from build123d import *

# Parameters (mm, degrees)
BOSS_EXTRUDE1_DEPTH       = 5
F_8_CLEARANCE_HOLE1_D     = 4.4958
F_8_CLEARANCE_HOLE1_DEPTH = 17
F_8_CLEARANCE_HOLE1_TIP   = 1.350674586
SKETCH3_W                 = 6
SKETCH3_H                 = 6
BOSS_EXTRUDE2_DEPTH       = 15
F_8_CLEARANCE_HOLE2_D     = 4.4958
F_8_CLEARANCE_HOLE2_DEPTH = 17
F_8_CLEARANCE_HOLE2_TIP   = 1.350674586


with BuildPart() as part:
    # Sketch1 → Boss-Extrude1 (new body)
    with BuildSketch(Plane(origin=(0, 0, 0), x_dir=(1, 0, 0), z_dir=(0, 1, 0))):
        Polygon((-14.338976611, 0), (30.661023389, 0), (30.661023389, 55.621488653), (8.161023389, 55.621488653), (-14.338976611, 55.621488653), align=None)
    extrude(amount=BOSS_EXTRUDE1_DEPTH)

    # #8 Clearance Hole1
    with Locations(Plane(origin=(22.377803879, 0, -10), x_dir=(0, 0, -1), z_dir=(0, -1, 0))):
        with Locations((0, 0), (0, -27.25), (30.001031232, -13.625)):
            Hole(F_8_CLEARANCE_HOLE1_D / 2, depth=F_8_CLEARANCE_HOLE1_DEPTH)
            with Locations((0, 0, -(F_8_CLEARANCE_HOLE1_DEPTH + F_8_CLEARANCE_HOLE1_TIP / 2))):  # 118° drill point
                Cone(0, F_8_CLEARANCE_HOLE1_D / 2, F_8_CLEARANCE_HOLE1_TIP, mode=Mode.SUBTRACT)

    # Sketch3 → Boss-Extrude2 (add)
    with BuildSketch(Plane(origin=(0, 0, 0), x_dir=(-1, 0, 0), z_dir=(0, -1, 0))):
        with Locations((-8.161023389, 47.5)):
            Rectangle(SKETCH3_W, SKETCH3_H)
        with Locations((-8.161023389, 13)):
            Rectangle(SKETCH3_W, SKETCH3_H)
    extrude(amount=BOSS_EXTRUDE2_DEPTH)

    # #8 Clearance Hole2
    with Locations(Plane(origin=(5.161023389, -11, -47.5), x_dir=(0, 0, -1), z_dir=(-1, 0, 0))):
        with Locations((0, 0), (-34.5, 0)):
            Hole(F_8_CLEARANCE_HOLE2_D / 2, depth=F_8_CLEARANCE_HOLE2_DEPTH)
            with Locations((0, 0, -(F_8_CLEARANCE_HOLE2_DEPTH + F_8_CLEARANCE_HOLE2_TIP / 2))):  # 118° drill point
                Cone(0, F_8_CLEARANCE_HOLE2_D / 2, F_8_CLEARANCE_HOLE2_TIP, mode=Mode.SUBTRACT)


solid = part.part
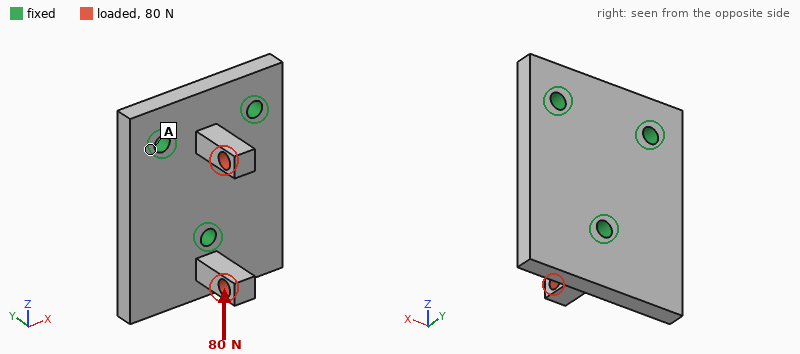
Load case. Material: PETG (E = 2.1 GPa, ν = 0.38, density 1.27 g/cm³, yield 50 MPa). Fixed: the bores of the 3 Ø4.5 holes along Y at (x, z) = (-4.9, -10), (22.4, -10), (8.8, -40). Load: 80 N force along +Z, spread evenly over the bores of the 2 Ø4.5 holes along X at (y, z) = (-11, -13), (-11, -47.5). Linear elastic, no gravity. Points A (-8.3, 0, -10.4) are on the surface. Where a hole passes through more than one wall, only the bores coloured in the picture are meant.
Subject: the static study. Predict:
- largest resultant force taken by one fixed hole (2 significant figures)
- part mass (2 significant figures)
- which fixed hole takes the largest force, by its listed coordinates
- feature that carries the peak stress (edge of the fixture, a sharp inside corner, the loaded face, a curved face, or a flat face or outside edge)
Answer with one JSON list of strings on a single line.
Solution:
["52 N", "17 g", "(8.8, -40)", "a flat face or outside edge"]
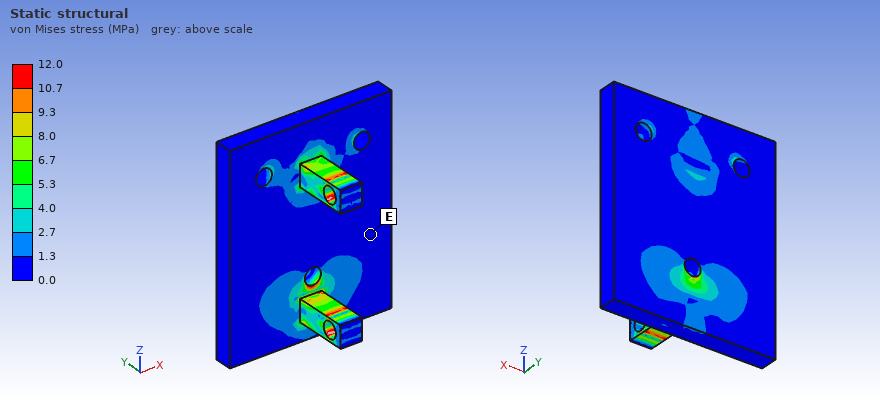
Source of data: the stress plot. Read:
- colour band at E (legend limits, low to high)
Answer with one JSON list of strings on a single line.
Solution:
["0.0 to 1.3 MPa"]
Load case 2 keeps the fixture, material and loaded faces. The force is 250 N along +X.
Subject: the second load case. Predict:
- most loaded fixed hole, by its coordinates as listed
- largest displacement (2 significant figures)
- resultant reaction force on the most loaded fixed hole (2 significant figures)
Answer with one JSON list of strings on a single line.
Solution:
["(8.8, -40)", "0.88 mm", "140 N"]
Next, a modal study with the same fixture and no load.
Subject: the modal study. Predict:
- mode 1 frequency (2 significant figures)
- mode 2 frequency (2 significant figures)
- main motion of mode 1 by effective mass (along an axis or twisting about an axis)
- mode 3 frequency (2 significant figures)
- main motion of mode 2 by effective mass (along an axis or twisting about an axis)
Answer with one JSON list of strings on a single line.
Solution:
["1900 Hz", "2300 Hz", "twisting about Z", "3100 Hz", "along Y"]
